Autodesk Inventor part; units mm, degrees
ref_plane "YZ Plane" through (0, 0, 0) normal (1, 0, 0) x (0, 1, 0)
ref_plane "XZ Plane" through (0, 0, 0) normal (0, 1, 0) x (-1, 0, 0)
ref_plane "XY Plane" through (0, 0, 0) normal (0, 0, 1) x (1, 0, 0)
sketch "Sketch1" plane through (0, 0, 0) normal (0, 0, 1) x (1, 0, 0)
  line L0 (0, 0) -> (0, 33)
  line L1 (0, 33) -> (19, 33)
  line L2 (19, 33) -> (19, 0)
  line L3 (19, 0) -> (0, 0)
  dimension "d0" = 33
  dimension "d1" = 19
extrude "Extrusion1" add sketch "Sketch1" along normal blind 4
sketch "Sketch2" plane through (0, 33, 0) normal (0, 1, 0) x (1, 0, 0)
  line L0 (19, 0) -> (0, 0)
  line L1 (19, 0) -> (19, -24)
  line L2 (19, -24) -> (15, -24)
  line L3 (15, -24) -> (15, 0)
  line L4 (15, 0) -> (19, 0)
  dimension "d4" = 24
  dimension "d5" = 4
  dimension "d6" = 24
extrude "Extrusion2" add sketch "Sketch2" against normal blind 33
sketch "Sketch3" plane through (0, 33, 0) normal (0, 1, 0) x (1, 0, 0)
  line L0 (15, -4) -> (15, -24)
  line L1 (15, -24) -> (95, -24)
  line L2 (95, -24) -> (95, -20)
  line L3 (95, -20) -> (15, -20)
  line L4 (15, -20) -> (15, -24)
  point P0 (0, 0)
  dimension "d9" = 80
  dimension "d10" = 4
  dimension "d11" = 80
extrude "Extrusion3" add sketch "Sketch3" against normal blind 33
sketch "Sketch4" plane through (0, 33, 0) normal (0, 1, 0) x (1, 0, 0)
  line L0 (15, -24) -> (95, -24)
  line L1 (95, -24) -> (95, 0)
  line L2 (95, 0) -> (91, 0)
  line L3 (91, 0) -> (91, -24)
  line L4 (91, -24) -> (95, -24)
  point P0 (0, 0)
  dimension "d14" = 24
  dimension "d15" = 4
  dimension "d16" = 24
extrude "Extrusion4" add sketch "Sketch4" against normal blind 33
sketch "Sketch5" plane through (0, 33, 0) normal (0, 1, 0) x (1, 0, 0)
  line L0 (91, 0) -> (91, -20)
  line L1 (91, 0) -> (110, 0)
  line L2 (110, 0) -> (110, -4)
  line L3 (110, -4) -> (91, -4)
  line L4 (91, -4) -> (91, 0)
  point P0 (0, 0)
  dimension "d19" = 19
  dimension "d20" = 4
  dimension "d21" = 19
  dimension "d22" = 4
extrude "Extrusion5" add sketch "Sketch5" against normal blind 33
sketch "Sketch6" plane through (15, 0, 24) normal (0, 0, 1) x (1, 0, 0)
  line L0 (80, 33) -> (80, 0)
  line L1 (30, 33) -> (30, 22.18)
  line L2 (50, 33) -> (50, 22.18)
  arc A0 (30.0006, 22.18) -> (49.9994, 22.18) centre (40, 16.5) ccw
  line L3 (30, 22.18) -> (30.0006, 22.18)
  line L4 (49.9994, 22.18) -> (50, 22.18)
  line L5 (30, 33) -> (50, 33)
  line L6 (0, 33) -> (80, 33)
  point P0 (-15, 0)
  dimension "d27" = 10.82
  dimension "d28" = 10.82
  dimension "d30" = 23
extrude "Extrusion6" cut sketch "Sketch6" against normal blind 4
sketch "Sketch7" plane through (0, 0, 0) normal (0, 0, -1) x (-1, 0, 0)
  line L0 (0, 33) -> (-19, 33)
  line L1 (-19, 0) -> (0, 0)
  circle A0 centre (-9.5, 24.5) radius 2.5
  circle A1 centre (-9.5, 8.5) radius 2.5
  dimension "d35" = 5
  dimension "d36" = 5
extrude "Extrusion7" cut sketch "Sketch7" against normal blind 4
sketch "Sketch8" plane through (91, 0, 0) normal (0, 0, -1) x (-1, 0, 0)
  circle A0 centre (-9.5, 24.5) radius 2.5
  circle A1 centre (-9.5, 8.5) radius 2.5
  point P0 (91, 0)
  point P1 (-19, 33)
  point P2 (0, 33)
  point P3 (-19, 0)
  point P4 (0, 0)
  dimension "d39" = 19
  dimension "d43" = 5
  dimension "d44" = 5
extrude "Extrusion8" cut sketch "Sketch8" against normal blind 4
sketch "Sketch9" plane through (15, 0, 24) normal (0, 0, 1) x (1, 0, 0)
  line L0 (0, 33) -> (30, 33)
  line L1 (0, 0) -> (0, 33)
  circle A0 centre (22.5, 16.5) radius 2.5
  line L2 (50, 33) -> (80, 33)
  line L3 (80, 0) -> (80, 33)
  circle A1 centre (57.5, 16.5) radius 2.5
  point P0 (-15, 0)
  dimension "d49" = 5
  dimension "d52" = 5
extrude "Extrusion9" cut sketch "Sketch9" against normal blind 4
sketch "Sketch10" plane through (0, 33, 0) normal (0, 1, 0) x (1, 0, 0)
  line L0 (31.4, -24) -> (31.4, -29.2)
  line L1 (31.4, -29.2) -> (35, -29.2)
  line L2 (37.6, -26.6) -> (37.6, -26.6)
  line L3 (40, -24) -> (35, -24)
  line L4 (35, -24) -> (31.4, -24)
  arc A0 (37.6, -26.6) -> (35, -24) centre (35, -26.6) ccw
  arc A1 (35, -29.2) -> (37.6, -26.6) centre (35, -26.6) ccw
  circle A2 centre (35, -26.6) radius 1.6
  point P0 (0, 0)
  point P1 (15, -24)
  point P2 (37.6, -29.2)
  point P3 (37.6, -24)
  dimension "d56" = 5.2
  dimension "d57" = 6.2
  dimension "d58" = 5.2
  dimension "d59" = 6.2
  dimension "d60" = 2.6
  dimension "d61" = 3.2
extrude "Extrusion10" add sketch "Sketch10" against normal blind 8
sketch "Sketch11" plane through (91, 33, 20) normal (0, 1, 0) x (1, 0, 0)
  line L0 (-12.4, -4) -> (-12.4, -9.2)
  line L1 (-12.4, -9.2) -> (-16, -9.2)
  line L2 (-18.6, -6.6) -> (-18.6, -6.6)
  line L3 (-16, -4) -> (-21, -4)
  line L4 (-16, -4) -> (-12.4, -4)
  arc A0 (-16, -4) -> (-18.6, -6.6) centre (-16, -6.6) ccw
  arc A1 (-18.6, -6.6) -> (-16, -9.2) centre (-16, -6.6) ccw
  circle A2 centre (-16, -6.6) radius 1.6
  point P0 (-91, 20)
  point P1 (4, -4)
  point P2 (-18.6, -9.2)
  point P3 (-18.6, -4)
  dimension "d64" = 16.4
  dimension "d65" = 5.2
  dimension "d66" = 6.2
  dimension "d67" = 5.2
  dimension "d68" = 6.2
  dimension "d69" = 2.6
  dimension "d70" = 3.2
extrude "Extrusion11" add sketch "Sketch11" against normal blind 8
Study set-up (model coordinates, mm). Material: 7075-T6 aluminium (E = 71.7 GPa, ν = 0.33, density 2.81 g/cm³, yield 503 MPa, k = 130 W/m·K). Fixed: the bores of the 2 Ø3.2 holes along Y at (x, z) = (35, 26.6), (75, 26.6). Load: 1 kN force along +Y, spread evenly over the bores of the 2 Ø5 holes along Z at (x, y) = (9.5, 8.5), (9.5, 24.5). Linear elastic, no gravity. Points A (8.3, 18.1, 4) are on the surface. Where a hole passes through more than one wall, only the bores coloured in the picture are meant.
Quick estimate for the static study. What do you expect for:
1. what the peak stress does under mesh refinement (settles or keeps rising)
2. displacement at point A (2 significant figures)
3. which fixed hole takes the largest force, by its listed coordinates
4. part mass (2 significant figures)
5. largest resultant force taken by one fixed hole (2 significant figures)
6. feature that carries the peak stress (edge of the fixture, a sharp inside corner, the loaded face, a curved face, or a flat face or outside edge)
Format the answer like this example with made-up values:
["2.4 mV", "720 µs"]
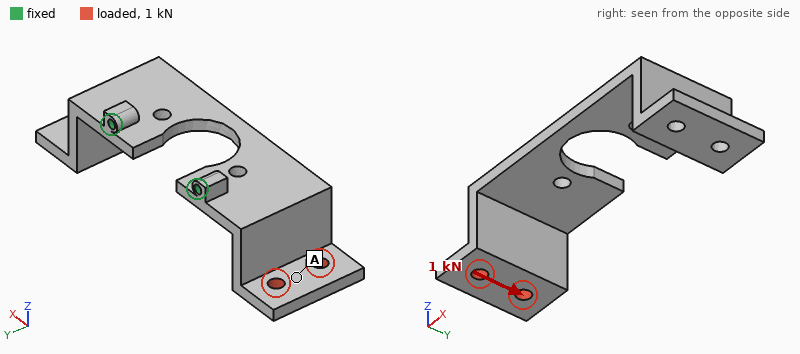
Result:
["keeps rising", "0.69 mm", "(35, 26.6)", "49 g", "1.3 kN", "edge of the fixture"]
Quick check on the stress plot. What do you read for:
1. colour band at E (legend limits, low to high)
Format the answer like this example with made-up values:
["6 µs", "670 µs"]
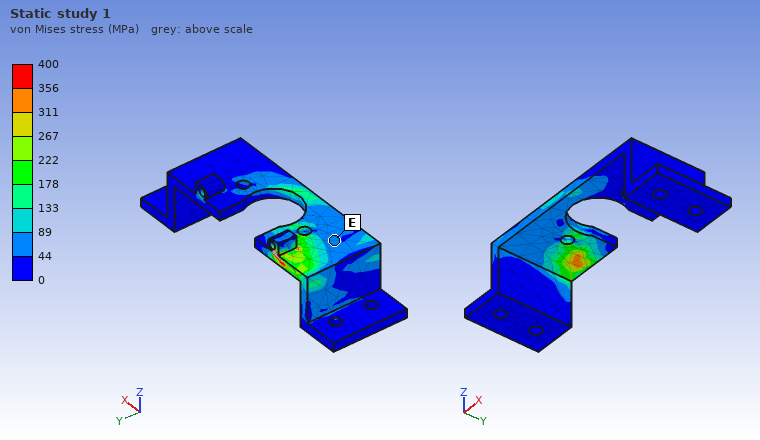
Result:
["44 to 89 MPa"]
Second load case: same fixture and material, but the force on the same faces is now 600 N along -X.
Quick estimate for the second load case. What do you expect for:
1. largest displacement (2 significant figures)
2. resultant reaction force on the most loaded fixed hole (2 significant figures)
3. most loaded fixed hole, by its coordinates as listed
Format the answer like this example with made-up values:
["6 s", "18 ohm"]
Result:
["1.3 mm", "440 N", "(35, 26.6)"]
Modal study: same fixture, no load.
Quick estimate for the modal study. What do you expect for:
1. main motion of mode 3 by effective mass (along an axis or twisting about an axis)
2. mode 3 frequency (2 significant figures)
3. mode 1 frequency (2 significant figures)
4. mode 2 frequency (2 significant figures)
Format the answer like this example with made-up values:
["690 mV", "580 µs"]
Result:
["along Y", "1700 Hz", "1100 Hz", "1100 Hz"]
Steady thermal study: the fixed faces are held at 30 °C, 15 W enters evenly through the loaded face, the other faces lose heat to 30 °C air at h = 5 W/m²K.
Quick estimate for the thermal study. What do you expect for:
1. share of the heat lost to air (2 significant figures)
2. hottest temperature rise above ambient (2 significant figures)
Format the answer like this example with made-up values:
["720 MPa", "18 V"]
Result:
["5.7 %", "52 K"]
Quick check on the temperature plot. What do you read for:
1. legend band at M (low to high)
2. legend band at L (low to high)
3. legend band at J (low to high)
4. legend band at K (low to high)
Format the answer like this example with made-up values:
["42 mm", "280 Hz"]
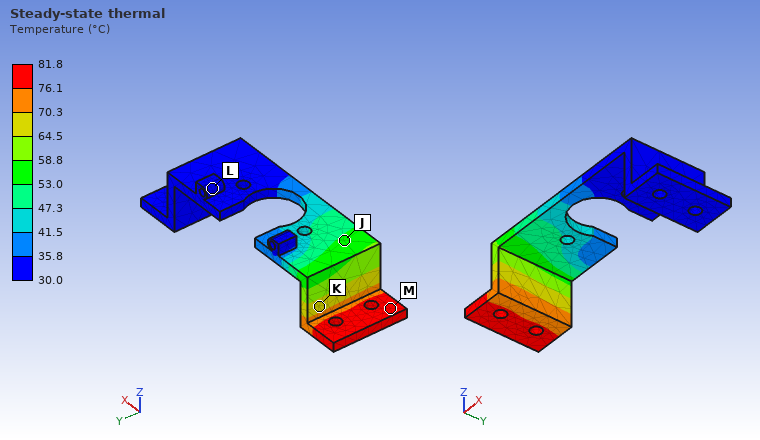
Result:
["76.1 to 81.8 °C", "30.0 to 35.8 °C", "53.0 to 58.8 °C", "64.5 to 70.3 °C"]
